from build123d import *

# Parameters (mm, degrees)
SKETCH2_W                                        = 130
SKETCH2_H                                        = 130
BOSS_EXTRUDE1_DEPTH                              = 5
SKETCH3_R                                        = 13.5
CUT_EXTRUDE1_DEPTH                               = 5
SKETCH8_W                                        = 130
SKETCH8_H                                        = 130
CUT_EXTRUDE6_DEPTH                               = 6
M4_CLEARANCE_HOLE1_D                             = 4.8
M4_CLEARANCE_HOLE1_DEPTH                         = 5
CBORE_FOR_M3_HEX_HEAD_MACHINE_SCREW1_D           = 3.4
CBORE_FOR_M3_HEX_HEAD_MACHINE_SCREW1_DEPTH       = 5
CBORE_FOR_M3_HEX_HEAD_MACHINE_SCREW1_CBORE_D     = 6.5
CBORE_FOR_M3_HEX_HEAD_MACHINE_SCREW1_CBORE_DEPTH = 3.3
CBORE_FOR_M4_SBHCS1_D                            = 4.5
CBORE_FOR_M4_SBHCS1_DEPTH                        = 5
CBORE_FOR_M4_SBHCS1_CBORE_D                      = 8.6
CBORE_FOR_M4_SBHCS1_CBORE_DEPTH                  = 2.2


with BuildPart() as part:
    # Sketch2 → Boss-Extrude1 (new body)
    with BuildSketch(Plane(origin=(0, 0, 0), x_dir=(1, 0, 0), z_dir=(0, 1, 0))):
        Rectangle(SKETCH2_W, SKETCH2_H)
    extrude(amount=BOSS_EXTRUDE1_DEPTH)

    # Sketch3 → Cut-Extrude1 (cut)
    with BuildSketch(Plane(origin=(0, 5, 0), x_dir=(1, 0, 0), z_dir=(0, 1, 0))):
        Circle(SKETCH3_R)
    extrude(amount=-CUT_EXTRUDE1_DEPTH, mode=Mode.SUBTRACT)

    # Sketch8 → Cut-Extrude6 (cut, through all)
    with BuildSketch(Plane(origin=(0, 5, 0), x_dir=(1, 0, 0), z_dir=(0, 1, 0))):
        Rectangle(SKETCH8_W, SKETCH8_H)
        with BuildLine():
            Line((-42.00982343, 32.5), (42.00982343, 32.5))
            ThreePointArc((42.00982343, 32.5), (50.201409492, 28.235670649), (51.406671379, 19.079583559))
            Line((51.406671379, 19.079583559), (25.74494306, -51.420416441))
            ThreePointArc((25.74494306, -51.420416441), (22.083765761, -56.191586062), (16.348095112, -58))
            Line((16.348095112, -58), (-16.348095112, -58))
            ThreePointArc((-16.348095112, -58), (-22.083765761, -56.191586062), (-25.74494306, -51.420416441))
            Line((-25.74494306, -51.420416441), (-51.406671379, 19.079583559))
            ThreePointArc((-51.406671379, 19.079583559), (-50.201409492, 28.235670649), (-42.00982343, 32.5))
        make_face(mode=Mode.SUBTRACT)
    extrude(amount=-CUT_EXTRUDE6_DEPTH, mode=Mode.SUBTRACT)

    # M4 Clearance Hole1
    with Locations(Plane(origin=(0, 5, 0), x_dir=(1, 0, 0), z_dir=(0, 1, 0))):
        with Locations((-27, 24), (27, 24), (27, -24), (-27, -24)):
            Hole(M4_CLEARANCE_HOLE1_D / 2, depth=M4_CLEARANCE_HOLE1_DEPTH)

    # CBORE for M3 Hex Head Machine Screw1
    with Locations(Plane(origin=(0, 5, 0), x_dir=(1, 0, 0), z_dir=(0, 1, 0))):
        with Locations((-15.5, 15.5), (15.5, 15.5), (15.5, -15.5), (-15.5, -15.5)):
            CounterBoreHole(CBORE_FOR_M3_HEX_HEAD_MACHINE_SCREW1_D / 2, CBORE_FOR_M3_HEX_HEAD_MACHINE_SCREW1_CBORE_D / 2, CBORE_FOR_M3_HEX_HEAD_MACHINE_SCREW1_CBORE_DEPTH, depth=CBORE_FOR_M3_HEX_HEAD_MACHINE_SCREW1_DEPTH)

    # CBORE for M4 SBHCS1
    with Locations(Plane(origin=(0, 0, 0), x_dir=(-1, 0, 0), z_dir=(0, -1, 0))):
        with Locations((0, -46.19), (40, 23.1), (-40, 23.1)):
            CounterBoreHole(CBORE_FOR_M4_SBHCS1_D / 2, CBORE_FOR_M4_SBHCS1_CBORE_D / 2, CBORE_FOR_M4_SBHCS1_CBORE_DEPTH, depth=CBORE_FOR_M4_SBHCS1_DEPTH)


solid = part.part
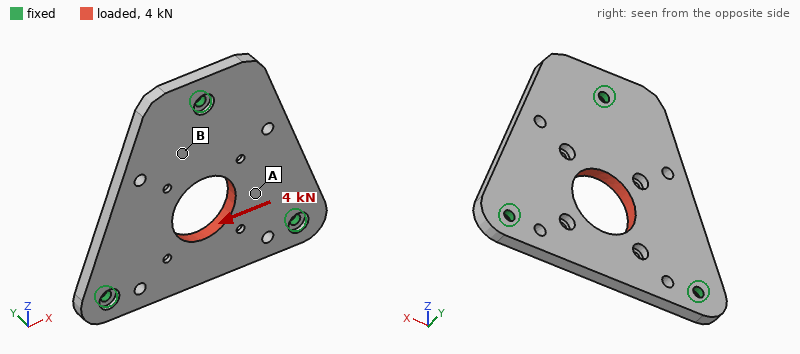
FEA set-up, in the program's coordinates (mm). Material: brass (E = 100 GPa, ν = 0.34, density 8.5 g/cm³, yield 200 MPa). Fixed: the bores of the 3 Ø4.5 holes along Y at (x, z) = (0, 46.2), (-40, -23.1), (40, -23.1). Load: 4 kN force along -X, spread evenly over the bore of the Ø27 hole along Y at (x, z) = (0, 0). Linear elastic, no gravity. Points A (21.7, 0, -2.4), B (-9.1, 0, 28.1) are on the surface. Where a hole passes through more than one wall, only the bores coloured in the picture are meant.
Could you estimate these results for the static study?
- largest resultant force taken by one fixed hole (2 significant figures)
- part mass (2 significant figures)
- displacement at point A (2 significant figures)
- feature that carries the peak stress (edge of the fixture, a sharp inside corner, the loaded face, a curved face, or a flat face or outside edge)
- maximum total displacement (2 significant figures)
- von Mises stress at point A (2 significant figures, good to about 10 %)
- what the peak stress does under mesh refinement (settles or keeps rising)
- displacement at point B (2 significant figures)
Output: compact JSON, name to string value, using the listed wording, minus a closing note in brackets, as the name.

{"largest resultant force taken by one fixed hole": "1.4 kN", "part mass": "270 g", "displacement at point A": "7.8 µm", "feature that carries the peak stress": "edge of the fixture", "maximum total displacement": "10 µm", "von Mises stress at point A": "12 MPa", "what the peak stress does under mesh refinement": "keeps rising", "displacement at point B": "6.7 µm"}
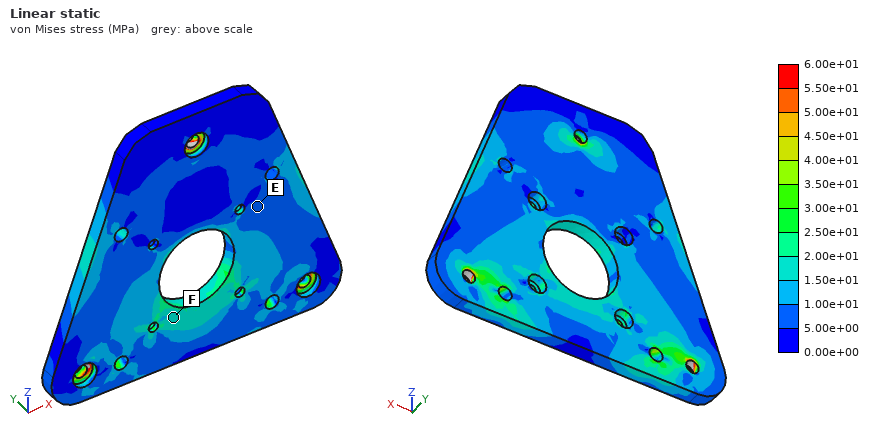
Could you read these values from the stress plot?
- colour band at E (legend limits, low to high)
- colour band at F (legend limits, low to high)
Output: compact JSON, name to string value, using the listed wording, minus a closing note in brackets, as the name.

{"colour band at E": "5.00e+00 to 1.00e+01 MPa", "colour band at F": "1.50e+01 to 2.00e+01 MPa"}
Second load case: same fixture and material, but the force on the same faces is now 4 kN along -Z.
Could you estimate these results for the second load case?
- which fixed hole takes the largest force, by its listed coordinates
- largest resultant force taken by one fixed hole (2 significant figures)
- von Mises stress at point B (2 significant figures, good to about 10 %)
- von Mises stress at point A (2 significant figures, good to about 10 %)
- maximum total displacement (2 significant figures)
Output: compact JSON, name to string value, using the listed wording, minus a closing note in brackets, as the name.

{"which fixed hole takes the largest force, by its listed coordinates": "(0, 46.2)", "largest resultant force taken by one fixed hole": "1.7 kN", "von Mises stress at point B": "12 MPa", "von Mises stress at point A": "8.3 MPa", "maximum total displacement": "13 µm"}
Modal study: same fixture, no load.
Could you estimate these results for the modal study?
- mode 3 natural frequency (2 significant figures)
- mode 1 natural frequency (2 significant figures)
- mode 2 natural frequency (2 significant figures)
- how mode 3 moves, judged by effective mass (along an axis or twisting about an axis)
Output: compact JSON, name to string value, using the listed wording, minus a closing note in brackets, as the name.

{"mode 3 natural frequency": "2500 Hz", "mode 1 natural frequency": "1900 Hz", "mode 2 natural frequency": "2000 Hz", "how mode 3 moves, judged by effective mass": "twisting about X"}
